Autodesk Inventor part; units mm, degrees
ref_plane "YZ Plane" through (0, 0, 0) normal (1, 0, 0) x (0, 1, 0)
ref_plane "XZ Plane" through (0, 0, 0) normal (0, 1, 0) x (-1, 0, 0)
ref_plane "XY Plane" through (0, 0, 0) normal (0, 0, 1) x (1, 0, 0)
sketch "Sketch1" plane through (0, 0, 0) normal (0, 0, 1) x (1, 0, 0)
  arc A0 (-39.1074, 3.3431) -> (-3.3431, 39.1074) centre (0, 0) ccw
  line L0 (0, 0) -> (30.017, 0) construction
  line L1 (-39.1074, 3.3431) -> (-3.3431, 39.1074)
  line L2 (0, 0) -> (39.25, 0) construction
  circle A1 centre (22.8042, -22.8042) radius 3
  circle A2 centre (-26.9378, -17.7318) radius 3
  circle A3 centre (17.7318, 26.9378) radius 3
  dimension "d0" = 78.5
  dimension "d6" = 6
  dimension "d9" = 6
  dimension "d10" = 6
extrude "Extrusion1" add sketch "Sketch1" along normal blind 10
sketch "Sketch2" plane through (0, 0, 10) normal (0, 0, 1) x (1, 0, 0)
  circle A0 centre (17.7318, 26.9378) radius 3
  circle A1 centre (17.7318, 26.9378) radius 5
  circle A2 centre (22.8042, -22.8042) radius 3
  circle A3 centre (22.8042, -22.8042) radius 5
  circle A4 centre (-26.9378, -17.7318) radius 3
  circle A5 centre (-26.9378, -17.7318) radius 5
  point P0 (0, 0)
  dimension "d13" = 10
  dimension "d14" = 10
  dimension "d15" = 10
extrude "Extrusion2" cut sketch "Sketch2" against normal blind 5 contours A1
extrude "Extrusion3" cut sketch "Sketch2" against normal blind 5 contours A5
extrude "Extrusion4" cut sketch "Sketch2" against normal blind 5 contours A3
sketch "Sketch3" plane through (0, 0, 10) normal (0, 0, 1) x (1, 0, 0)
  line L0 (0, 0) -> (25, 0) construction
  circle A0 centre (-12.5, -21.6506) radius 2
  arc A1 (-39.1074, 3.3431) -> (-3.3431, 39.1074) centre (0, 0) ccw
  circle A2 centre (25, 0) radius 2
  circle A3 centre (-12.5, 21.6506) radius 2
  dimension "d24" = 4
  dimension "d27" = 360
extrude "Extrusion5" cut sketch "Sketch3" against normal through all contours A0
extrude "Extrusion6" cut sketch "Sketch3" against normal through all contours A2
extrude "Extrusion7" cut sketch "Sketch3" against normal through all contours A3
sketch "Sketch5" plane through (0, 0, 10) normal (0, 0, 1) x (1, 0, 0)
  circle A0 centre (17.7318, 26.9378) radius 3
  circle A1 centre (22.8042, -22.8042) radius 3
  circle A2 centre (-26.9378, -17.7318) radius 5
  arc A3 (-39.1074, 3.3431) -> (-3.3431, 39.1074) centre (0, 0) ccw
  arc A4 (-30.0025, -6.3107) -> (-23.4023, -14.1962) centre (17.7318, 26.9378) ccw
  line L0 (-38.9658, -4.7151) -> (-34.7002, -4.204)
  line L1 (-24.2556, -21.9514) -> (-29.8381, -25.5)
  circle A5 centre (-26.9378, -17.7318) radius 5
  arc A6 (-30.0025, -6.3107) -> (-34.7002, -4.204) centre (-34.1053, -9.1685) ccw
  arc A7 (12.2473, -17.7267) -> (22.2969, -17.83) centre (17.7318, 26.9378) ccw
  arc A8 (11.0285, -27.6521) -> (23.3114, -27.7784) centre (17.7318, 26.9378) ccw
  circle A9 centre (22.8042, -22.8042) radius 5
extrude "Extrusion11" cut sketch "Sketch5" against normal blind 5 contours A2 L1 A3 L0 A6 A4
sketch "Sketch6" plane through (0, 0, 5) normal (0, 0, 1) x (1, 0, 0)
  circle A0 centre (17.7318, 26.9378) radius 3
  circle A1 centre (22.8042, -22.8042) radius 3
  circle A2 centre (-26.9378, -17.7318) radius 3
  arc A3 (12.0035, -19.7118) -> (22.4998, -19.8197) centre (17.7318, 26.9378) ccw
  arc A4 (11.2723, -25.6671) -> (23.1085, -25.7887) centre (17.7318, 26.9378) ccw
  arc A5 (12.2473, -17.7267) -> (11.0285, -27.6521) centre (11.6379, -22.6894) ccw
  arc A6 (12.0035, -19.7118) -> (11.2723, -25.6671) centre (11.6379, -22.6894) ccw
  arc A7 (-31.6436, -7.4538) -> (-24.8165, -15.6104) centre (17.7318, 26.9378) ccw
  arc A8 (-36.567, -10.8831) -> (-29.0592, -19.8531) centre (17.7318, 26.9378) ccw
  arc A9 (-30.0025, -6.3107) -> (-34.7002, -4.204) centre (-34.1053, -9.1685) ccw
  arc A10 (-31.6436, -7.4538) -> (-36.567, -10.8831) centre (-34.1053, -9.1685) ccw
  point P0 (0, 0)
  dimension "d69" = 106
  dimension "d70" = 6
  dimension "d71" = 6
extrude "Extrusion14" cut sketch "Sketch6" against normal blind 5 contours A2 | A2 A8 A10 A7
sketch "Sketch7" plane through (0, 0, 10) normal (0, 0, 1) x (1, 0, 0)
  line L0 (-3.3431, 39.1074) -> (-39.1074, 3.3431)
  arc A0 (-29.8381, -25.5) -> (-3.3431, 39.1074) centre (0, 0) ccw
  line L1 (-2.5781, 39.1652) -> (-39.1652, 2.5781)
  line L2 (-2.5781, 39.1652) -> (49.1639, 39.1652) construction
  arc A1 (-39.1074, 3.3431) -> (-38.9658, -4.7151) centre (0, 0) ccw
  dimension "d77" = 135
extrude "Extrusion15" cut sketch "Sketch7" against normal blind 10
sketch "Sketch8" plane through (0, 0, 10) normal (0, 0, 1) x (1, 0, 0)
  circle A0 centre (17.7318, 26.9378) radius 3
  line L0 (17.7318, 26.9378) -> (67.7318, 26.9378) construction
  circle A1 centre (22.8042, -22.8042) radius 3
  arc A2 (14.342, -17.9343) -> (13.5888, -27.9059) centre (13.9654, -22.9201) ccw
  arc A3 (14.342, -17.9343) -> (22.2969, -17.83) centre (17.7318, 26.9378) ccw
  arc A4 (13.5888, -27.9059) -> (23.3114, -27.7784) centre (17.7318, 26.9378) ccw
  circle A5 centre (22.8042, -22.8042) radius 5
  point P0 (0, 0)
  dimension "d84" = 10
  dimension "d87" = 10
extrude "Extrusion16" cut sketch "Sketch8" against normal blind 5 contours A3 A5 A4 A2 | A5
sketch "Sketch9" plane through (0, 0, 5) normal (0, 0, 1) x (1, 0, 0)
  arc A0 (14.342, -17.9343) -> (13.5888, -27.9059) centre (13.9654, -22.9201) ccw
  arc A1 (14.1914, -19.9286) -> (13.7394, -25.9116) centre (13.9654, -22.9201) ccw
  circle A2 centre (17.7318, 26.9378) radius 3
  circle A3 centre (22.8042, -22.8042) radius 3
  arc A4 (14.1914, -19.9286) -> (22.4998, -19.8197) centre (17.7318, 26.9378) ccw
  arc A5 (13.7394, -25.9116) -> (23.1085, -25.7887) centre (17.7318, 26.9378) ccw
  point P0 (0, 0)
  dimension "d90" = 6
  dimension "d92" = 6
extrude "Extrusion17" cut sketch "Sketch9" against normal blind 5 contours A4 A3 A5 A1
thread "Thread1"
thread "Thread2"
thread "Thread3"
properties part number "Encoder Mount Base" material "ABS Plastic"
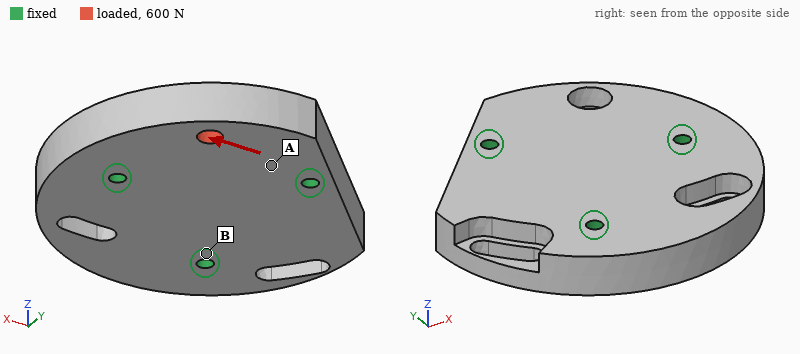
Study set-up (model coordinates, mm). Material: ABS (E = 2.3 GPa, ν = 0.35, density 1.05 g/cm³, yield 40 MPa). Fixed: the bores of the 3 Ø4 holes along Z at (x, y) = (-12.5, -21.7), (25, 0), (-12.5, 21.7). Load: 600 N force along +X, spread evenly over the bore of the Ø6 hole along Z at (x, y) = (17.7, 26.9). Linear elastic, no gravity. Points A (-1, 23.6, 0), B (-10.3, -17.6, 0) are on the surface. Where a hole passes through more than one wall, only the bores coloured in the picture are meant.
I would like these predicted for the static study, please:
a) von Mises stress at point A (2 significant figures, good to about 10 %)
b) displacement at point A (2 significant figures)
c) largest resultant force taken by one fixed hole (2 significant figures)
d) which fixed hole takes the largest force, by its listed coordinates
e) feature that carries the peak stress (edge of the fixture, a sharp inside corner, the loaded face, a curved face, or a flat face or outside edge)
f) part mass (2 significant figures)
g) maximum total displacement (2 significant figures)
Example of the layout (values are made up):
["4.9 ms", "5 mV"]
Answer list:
["3.7 MPa", "17 µm", "430 N", "(-12.5, 21.7)", "the loaded face", "43 g", "81 µm"]
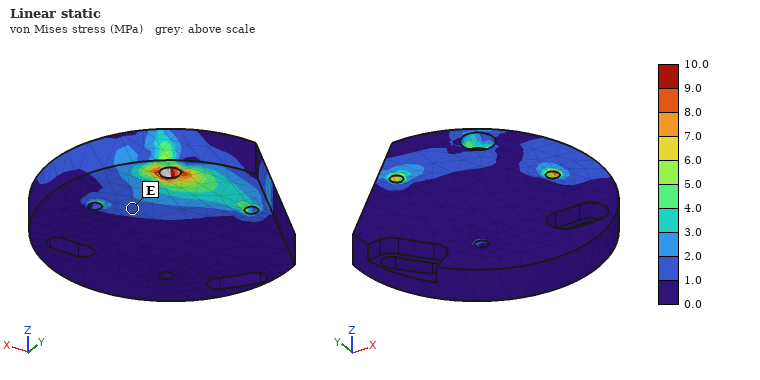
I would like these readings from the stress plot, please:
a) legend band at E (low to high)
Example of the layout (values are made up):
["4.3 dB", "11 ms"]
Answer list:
["1.0 to 2.0 MPa"]
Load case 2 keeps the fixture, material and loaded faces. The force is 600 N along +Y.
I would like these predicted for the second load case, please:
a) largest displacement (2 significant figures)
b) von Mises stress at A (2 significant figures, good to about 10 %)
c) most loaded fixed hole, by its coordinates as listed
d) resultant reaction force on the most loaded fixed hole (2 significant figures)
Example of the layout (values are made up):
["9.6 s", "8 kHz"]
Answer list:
["0.10 mm", "1.9 MPa", "(25, 0)", "430 N"]
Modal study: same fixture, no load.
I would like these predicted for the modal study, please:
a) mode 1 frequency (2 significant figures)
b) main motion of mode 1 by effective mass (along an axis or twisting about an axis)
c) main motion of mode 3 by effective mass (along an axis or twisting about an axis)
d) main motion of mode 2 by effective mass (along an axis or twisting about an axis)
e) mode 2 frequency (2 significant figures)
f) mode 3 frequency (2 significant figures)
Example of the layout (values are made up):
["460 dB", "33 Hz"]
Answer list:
["2800 Hz", "twisting about X", "along Z", "twisting about Y", "2900 Hz", "3500 Hz"]
